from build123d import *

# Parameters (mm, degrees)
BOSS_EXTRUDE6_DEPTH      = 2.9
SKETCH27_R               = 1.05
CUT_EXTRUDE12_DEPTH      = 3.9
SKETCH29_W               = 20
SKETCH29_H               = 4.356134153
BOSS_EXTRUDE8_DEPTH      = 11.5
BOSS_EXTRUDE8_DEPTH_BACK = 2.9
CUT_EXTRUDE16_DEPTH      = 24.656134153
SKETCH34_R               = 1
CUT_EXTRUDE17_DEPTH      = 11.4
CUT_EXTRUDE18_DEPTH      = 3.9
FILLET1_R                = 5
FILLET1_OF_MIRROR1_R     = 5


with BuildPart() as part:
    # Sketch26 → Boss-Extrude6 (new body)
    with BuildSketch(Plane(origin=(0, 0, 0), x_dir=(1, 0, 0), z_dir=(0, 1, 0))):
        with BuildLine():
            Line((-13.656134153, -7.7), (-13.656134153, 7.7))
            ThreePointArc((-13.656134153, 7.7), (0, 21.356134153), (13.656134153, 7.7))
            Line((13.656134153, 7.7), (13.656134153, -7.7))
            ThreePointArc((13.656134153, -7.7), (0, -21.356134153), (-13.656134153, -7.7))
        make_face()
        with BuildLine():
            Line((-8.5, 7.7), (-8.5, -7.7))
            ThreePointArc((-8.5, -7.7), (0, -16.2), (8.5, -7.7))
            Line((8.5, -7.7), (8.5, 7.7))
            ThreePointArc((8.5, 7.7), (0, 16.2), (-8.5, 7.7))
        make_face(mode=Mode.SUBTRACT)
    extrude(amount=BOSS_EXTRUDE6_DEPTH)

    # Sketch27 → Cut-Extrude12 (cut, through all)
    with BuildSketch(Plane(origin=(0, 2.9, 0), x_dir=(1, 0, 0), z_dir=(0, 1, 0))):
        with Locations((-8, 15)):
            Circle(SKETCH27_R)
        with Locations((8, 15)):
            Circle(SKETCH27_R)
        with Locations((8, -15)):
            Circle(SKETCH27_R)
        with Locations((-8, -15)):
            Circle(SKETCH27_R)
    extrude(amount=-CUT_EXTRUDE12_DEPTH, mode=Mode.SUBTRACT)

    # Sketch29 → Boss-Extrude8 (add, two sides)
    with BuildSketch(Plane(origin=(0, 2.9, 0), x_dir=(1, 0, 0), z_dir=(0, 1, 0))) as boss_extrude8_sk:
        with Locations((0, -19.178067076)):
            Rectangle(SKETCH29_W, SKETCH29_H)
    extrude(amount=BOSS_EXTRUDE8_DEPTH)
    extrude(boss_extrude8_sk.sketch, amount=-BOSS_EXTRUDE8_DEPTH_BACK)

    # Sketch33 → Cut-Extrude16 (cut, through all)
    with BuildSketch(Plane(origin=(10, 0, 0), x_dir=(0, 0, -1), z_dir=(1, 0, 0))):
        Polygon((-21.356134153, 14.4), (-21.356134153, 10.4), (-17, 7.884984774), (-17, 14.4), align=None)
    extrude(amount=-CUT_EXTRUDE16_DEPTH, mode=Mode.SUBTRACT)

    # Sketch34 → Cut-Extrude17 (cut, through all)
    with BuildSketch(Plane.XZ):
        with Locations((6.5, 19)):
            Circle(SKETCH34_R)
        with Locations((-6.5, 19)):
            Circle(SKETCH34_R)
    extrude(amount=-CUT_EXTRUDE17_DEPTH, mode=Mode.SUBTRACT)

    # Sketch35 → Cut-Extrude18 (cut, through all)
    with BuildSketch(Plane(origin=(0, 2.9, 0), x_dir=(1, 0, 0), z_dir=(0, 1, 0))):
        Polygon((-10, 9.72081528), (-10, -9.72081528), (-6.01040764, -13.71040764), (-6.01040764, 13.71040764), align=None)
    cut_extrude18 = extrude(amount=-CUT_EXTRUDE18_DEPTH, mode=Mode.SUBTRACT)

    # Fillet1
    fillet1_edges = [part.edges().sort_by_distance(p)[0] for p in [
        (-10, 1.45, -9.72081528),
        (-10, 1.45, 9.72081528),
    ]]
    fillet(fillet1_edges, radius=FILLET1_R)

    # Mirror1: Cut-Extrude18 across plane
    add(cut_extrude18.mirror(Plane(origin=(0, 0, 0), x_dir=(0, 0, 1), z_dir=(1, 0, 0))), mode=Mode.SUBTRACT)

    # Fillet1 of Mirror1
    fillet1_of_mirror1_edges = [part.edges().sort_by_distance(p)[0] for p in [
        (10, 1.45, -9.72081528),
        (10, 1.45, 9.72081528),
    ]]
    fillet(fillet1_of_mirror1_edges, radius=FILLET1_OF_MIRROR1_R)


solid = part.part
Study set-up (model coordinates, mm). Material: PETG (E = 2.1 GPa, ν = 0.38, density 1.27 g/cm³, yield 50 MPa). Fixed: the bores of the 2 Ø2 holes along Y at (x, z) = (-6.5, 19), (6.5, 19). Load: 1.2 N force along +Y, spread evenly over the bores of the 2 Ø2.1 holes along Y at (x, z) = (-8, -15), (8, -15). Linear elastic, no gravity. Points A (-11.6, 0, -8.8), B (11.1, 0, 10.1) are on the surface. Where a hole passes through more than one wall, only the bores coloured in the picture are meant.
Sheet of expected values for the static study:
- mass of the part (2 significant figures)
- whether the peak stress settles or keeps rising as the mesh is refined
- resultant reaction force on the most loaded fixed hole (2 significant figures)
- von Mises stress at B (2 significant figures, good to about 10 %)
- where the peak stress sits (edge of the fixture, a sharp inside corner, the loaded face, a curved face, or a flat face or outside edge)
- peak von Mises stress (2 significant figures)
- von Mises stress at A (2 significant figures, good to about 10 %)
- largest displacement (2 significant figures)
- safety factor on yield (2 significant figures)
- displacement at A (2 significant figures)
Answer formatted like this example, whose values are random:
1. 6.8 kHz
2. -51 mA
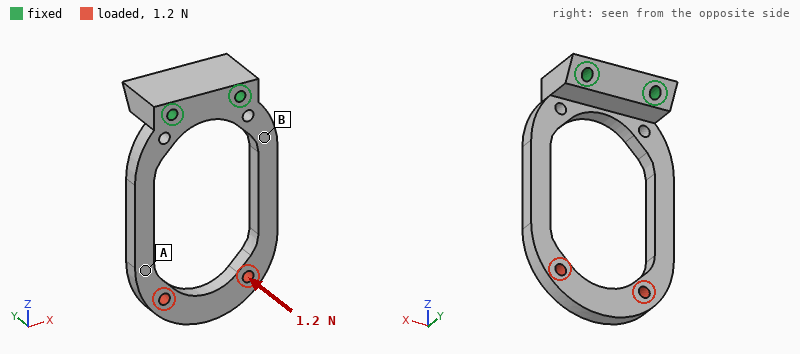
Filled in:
1. 2.3 g
2. settles
3. 0.60 N
4. 2.8 MPa
5. a curved face
6. 6.3 MPa
7. 0.70 MPa
8. 0.61 mm
9. 7.9
10. 0.34 mm
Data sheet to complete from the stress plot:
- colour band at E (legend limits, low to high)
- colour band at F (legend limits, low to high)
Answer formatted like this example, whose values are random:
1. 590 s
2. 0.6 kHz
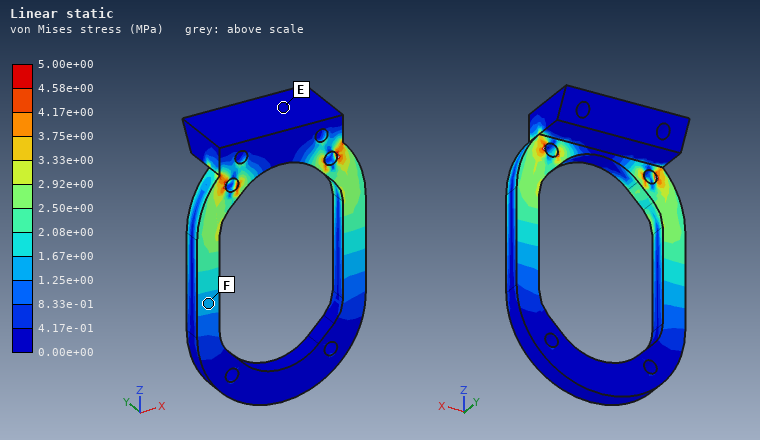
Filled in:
1. 0.00e+00 to 4.17e-01 MPa
2. 1.25e+00 to 1.67e+00 MPa
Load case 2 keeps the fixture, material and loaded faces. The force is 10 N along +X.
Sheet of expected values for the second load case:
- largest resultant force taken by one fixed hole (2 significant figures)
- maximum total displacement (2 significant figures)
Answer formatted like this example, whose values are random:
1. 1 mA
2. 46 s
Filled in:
1. 19 N
2. 0.53 mm
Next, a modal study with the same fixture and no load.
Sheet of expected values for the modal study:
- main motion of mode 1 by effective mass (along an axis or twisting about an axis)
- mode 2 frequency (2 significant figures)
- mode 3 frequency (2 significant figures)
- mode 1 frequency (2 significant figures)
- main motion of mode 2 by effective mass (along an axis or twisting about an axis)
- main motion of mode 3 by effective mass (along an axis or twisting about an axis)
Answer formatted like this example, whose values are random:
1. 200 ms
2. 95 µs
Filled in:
1. along Y
2. 820 Hz
3. 890 Hz
4. 300 Hz
5. along X
6. twisting about Z
